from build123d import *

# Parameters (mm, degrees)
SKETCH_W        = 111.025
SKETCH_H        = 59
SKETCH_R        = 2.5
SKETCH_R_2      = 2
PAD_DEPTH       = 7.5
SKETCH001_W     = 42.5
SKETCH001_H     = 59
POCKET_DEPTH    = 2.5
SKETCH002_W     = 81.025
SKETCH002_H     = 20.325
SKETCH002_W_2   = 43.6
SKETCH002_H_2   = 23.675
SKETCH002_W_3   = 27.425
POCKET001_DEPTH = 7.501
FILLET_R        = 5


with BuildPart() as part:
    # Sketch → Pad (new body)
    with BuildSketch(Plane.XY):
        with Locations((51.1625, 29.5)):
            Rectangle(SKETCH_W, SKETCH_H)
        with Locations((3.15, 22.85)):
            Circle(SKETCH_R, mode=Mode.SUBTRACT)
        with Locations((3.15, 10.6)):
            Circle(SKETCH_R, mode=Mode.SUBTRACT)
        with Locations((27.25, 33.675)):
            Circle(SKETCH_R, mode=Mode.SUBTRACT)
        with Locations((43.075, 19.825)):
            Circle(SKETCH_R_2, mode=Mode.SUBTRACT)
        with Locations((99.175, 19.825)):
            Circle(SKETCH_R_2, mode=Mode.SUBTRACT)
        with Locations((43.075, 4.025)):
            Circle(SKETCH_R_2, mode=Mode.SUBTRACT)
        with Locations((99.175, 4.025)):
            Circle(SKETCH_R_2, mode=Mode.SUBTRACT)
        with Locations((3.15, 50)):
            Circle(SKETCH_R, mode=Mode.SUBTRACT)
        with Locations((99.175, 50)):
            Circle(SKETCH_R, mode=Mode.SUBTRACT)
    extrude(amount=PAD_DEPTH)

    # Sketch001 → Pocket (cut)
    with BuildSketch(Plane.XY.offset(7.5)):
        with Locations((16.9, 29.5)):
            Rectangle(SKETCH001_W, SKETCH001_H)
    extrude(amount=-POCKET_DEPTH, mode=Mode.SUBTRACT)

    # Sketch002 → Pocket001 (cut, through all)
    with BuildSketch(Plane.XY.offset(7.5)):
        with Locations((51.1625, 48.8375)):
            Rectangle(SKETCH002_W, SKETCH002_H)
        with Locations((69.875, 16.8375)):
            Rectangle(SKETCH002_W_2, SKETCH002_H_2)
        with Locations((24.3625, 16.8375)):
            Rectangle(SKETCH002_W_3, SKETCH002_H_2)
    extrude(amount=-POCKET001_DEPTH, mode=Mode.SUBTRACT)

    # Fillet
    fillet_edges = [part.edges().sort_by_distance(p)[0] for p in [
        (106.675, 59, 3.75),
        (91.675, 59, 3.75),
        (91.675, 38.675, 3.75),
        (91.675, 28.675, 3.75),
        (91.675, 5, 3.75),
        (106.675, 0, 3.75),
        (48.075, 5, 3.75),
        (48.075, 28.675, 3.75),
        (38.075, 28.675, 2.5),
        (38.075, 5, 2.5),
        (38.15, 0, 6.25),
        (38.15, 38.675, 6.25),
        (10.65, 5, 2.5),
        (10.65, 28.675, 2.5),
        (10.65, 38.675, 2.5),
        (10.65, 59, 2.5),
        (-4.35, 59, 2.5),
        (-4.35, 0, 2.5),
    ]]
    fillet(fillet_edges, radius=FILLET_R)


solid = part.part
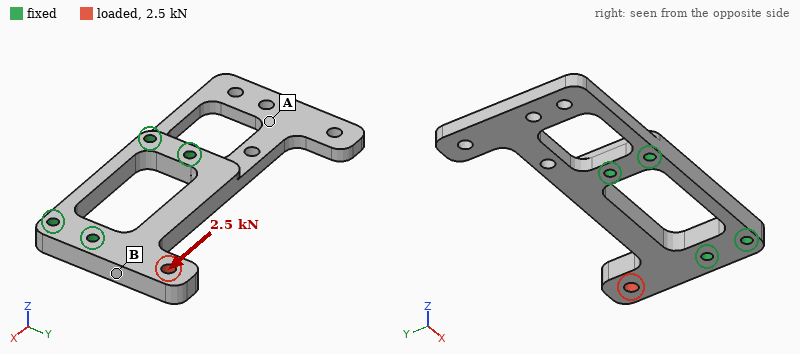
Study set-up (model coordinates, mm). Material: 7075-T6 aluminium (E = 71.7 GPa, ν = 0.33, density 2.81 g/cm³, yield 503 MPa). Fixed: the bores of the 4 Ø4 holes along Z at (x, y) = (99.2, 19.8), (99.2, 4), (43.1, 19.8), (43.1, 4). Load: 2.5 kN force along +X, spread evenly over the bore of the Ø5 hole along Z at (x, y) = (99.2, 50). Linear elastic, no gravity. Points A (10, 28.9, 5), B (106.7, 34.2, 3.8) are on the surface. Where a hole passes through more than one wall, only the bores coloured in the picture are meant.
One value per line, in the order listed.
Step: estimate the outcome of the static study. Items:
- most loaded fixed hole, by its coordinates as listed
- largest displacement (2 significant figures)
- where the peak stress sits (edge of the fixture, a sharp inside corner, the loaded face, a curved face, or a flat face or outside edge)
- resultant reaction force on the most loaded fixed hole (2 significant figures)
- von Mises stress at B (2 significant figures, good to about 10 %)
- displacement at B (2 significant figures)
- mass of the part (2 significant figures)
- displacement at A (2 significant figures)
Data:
(43.1, 19.8)
0.15 mm
a curved face
2.1 kN
79 MPa
0.043 mm
57 g
0.029 mm
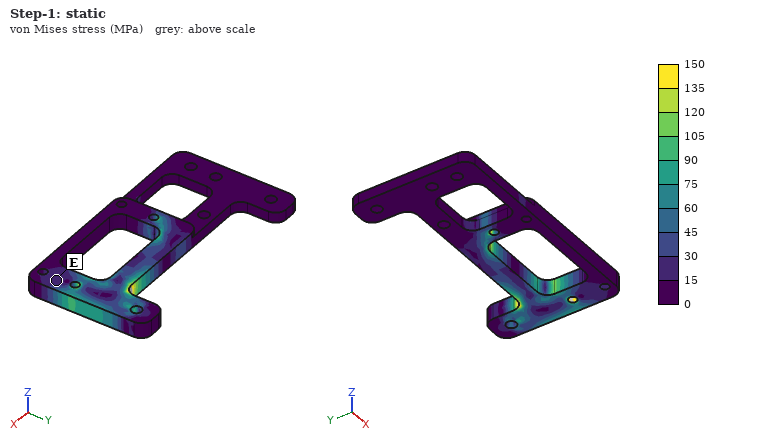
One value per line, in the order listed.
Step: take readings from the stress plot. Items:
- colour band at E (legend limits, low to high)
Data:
15 to 30 MPa
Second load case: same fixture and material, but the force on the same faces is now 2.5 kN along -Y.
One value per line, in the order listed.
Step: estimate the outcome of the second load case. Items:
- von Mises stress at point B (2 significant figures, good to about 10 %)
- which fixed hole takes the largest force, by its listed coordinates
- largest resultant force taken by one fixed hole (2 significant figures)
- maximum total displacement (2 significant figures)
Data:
26 MPa
(99.2, 19.8)
2.2 kN
13 µm
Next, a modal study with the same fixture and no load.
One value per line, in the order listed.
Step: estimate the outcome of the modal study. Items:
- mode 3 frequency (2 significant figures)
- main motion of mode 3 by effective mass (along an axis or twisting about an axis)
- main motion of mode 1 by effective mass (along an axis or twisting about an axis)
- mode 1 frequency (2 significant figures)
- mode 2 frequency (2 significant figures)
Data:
3300 Hz
along Y
along Z
1000 Hz
2200 Hz
